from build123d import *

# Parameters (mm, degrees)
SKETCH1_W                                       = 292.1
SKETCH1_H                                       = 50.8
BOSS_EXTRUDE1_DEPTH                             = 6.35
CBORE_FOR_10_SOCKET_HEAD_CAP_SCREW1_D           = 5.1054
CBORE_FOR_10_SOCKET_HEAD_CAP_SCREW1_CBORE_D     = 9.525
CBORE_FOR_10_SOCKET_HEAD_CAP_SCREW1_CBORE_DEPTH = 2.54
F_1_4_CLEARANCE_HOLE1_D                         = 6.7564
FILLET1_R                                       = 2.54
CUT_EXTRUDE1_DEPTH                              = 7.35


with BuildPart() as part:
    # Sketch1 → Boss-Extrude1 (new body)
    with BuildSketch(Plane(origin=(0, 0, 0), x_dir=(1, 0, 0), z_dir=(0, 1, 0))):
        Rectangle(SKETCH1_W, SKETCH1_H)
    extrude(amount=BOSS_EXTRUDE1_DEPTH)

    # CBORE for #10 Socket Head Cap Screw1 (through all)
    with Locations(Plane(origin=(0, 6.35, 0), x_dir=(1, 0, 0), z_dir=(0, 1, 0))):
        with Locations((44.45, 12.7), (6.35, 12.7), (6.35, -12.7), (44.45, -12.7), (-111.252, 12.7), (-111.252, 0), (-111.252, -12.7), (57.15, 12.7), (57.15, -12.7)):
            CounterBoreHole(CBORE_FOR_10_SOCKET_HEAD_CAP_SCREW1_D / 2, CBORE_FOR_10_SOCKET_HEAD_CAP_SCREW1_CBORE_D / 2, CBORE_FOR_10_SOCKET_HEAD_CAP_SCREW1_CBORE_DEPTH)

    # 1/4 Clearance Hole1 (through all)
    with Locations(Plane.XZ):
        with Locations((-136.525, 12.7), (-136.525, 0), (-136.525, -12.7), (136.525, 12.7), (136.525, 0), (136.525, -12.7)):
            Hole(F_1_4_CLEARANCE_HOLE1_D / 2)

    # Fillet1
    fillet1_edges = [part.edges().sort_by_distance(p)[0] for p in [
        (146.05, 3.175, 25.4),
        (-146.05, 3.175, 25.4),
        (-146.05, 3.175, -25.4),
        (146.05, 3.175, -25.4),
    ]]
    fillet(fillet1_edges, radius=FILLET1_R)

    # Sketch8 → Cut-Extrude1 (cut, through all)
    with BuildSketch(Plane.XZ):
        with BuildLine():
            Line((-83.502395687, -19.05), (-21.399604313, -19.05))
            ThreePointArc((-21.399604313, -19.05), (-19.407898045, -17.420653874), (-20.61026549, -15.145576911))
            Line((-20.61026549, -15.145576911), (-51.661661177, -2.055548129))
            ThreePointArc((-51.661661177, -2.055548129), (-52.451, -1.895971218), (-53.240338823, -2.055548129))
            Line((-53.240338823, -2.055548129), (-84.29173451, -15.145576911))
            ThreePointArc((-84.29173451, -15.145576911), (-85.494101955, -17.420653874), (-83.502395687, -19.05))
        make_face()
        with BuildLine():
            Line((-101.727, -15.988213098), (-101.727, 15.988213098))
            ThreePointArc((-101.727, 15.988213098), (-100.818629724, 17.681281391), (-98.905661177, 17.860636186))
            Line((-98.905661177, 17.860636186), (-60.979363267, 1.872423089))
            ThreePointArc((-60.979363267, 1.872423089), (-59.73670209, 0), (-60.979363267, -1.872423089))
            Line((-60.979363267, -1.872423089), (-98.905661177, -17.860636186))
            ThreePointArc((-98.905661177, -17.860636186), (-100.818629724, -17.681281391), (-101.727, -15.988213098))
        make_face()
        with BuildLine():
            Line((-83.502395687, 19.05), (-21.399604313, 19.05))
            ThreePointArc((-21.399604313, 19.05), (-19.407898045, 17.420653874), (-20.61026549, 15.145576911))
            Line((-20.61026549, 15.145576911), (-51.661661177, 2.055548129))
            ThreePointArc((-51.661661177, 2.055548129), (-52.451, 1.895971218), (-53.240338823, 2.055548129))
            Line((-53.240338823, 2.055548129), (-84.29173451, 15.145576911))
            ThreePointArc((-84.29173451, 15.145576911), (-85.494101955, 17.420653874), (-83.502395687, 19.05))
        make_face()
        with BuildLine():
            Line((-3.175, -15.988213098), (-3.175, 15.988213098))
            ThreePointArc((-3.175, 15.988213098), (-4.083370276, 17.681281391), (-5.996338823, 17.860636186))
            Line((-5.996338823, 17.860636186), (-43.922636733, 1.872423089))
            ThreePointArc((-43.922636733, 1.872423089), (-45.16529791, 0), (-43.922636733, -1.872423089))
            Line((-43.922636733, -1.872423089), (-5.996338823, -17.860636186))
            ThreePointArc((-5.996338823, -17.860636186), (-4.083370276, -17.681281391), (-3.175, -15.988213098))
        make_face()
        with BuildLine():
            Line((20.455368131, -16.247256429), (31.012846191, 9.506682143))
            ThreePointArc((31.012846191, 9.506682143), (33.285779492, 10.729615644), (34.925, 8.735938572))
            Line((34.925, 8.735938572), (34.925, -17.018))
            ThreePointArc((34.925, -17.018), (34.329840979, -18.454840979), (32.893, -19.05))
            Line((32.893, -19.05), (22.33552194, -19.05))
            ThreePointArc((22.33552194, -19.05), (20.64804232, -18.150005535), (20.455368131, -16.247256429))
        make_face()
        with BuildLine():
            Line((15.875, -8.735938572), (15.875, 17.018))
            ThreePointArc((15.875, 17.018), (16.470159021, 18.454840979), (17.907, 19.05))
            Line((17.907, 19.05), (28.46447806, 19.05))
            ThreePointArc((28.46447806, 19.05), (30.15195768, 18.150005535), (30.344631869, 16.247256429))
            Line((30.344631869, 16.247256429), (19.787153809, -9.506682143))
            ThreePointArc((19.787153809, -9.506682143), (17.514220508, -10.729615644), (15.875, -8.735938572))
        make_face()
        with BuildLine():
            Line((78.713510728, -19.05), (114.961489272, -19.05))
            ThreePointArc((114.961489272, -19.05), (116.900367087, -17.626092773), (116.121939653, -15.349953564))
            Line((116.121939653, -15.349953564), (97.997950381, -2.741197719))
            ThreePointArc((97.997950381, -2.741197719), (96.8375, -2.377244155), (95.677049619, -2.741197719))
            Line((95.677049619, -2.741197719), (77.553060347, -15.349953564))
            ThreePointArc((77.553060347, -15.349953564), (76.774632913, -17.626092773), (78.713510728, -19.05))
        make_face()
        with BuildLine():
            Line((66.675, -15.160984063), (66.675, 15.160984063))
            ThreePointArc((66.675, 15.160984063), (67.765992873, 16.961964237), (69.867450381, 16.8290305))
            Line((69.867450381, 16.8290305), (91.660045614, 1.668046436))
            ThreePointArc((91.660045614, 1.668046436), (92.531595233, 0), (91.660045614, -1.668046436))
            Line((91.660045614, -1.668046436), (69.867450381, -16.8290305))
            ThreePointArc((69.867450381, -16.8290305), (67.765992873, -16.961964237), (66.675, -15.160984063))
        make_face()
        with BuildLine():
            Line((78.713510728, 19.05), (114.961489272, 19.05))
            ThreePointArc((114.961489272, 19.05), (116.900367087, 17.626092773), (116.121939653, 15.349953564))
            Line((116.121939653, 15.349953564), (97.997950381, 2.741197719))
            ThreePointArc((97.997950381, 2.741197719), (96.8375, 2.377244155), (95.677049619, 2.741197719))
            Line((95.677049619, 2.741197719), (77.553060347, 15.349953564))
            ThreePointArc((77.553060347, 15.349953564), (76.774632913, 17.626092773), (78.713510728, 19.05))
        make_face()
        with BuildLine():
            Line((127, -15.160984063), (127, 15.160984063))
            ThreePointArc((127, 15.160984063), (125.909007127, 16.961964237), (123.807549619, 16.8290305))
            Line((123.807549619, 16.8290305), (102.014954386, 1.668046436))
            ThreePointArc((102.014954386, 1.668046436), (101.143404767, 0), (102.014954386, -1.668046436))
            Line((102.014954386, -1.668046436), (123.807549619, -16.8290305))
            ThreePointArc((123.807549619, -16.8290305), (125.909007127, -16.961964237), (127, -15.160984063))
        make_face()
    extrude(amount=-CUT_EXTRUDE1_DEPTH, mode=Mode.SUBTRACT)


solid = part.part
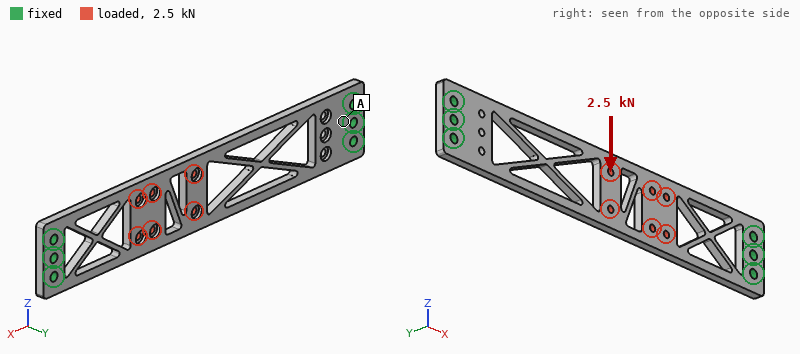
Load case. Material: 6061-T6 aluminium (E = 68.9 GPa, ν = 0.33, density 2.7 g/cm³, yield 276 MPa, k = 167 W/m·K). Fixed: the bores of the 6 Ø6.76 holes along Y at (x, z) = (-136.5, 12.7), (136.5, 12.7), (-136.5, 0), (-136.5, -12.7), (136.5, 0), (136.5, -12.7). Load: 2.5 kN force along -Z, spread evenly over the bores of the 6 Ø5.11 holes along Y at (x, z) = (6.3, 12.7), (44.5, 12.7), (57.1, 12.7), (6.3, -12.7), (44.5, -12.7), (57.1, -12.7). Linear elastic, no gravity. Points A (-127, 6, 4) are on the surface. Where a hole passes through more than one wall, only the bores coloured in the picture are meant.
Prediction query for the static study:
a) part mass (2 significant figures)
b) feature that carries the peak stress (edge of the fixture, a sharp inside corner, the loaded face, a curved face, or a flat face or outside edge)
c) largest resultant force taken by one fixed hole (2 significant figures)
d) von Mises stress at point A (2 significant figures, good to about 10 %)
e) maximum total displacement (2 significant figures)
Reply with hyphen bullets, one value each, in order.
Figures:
- 150 g
- a flat face or outside edge
- 2.4 kN
- 11 MPa
- 0.25 mm
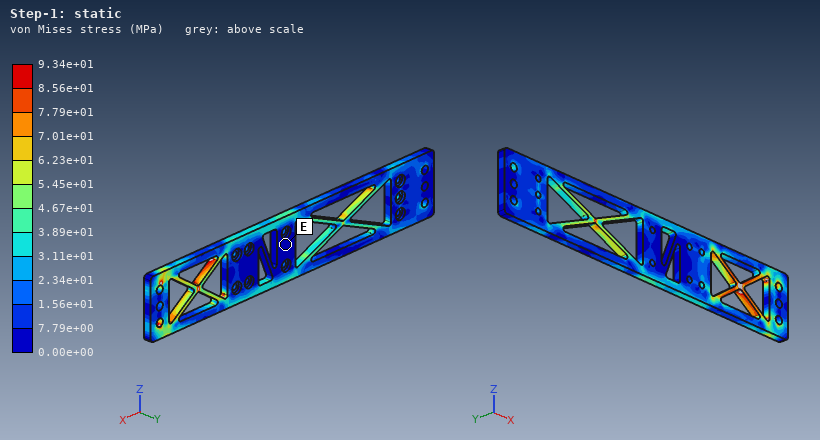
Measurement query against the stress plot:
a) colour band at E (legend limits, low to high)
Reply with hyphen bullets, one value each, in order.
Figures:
- 0.00e+00 to 7.79e+00 MPa
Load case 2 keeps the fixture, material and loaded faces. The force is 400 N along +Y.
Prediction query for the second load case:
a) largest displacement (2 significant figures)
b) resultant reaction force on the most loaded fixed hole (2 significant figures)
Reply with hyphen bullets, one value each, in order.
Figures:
- 1.1 mm
- 140 N
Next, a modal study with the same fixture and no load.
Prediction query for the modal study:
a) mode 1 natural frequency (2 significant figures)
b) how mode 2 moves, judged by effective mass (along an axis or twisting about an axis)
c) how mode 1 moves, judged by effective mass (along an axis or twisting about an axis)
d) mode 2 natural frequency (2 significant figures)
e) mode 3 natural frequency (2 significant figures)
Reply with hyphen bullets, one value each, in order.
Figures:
- 390 Hz
- twisting about X
- along Y
- 990 Hz
- 1200 Hz
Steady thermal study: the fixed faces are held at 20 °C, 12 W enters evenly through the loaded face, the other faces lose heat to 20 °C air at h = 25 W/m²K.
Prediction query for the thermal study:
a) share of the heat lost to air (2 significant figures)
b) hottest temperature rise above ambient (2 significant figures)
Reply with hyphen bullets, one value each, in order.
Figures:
- 52 %
- 18 K
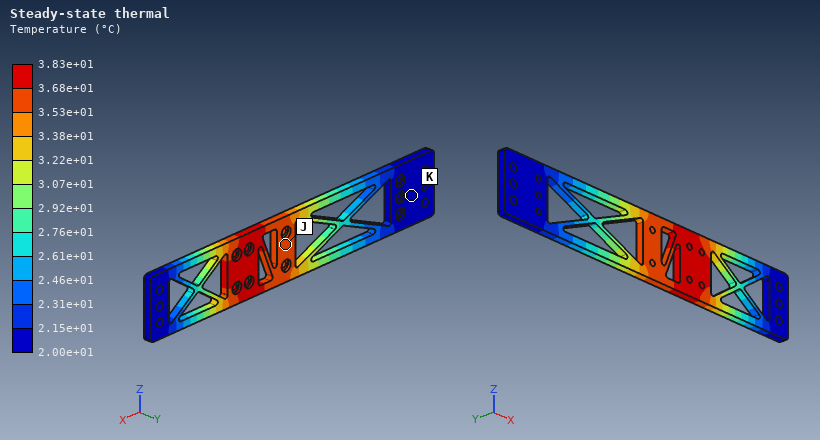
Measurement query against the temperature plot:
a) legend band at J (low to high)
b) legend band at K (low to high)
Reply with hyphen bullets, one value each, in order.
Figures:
- 3.53e+01 to 3.68e+01 °C
- 2.00e+01 to 2.15e+01 °C
